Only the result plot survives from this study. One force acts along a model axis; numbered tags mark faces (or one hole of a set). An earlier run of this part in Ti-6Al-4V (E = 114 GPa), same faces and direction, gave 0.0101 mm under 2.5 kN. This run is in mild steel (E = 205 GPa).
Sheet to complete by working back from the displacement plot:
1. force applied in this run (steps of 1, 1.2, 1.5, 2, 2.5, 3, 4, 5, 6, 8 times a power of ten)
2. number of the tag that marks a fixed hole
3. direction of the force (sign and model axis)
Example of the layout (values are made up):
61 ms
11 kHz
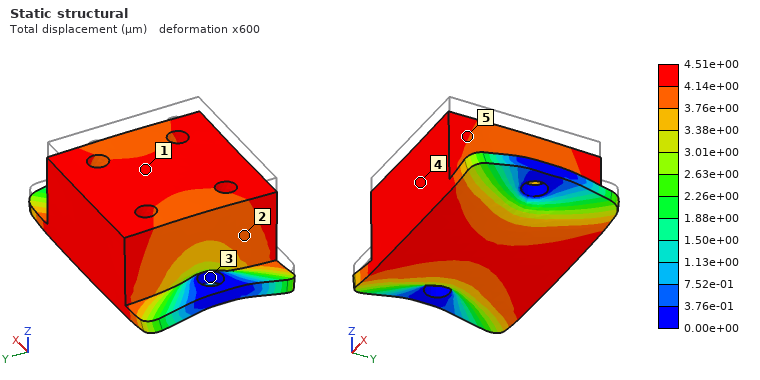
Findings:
2 kN
3
-Z
